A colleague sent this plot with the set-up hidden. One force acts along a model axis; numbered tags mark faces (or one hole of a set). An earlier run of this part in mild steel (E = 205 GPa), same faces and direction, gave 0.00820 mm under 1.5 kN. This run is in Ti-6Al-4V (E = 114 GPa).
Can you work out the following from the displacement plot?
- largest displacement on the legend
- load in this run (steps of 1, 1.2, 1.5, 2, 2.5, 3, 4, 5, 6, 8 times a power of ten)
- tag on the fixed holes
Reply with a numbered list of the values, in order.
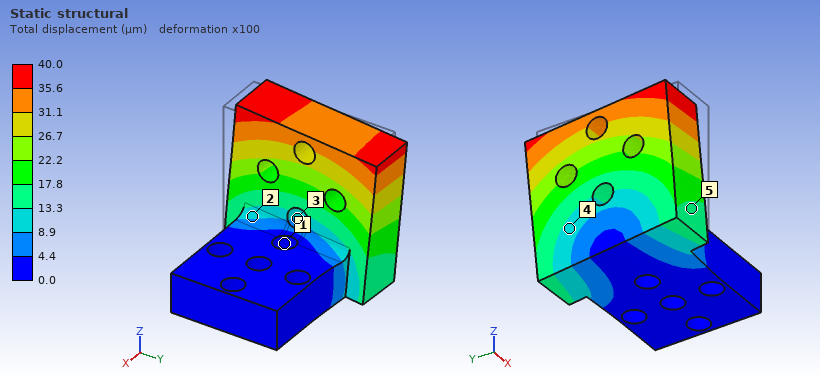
1. 40.0 µm
2. 4 kN
3. 1
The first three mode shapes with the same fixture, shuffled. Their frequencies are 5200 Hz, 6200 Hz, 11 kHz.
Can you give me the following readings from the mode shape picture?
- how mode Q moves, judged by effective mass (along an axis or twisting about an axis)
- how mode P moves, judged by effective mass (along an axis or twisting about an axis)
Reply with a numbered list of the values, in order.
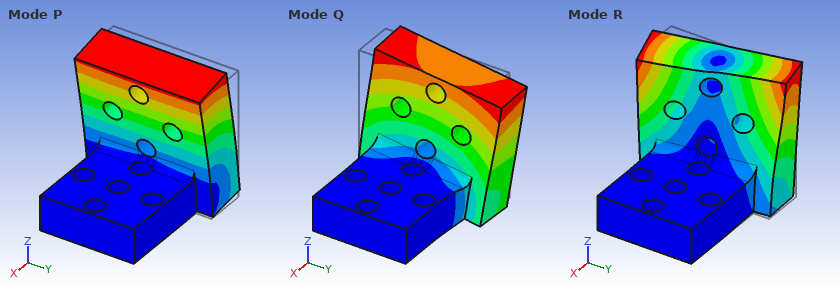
1. along Y
2. along X
